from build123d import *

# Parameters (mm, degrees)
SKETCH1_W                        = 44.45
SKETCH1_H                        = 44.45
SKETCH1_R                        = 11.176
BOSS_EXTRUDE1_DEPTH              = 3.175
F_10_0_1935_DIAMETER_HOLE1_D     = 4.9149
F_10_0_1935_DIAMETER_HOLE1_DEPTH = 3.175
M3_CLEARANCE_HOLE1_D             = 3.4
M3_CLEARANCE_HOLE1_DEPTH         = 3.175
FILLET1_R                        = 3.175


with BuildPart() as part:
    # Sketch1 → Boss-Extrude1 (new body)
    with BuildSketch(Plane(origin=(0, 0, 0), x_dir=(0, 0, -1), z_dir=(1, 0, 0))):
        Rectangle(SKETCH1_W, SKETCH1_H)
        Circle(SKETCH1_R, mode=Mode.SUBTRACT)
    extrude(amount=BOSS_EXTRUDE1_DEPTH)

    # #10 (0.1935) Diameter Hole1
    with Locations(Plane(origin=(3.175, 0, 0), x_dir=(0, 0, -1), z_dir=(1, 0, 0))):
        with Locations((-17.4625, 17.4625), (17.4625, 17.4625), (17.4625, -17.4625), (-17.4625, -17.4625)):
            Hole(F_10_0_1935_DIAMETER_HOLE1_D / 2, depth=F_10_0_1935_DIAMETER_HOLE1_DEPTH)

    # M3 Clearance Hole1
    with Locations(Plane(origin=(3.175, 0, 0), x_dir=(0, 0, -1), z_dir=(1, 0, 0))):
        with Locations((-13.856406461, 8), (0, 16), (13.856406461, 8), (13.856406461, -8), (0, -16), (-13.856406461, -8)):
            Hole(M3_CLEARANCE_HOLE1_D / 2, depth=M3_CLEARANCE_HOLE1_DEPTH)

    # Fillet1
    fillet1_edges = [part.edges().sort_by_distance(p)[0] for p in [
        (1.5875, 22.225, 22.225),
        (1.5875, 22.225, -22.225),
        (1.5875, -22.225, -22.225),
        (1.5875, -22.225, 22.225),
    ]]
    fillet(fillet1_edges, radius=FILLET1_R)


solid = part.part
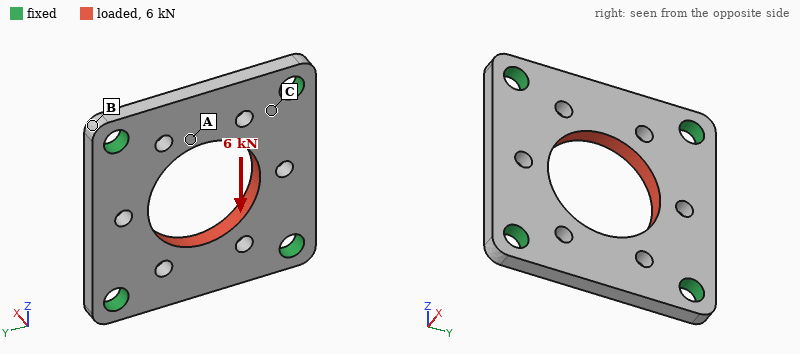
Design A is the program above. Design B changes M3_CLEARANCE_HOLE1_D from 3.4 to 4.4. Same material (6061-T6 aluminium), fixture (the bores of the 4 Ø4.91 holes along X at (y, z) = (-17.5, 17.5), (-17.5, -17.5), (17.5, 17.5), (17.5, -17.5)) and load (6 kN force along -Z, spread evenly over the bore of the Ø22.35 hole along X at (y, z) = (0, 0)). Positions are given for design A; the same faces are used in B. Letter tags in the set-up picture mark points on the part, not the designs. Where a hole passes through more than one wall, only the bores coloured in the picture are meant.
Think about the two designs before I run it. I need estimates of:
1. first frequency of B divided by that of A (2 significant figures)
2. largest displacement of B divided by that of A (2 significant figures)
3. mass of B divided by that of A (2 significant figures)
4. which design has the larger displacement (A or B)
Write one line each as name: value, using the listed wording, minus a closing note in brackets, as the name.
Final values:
first frequency of B divided by that of A: 1.0
largest displacement of B divided by that of A: 1.1
mass of B divided by that of A: 0.97
which design has the larger displacement: B
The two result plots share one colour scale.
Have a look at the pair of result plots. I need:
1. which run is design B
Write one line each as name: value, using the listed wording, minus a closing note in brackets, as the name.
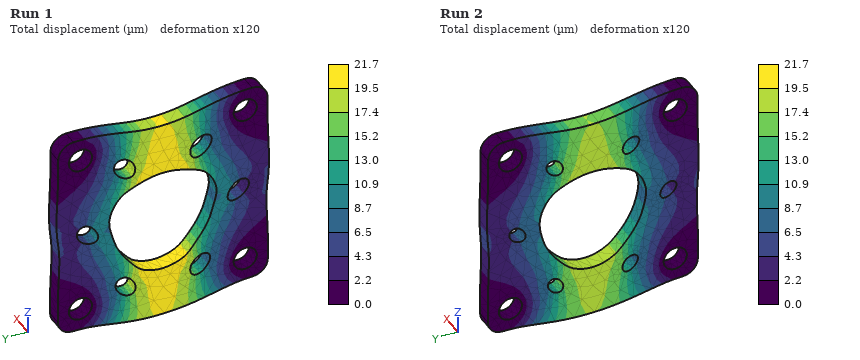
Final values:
which run is design B: Run 1
